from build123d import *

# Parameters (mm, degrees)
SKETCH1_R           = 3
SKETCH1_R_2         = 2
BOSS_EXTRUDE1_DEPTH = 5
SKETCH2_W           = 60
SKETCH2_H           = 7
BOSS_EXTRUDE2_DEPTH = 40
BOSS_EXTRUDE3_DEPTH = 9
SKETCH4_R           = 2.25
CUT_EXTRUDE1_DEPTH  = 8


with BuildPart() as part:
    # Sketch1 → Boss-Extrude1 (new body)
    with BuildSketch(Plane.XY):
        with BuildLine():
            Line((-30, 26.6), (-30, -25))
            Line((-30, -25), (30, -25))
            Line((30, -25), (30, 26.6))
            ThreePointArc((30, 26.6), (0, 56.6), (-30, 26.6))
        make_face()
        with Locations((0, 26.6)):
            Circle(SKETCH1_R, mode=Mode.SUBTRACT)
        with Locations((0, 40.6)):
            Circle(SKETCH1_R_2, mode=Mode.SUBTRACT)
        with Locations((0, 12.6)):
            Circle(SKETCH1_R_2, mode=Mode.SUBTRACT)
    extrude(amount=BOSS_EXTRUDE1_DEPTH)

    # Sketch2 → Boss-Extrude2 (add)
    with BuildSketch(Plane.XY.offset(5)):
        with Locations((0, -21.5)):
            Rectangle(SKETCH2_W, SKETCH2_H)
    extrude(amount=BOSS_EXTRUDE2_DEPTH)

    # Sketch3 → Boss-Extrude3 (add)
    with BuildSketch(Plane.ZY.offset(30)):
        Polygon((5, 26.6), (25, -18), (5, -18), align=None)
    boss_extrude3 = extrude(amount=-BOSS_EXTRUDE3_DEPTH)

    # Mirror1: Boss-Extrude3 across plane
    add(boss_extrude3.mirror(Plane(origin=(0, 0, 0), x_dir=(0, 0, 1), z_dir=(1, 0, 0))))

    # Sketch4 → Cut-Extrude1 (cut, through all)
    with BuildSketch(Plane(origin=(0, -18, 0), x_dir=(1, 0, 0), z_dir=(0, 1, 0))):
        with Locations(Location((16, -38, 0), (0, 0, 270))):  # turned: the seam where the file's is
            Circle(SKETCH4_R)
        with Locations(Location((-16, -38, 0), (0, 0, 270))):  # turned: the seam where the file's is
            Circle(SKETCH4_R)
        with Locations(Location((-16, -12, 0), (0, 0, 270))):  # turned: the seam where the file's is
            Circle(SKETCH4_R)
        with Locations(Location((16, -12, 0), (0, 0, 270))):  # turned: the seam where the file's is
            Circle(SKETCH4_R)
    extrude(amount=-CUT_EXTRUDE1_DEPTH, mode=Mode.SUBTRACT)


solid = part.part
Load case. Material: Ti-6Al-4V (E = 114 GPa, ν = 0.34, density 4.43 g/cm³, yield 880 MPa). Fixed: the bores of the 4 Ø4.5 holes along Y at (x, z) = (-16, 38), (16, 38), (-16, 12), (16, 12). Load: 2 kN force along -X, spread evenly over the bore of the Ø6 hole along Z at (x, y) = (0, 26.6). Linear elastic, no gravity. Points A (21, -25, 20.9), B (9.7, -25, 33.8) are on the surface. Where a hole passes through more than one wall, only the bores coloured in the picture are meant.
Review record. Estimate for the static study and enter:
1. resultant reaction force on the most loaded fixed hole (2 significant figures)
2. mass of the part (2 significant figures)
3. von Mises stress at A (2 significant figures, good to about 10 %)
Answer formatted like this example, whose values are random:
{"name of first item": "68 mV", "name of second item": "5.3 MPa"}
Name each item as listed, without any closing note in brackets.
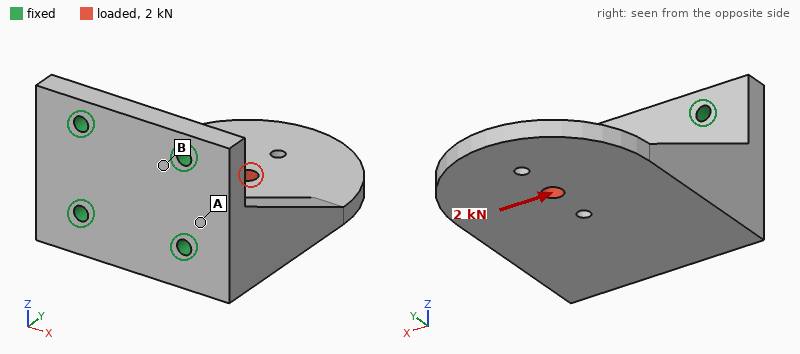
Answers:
{"resultant reaction force on the most loaded fixed hole": "2.8 kN", "mass of the part": "210 g", "von Mises stress at A": "25 MPa"}
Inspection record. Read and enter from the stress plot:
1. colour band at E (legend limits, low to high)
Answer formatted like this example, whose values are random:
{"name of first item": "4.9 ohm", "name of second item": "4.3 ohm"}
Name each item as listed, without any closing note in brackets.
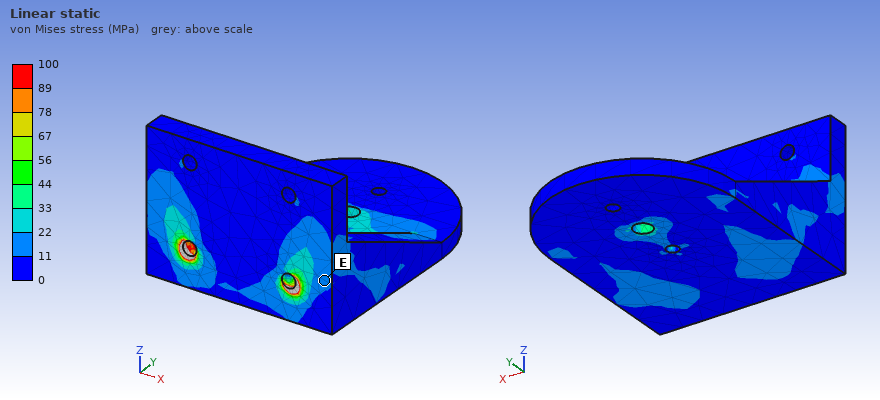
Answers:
{"colour band at E": "11 to 22 MPa"}
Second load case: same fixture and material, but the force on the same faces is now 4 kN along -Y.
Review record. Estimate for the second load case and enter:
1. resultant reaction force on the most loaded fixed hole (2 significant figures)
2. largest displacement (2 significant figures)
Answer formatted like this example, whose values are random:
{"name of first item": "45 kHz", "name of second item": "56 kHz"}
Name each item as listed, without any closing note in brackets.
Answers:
{"resultant reaction force on the most loaded fixed hole": "2.4 kN", "largest displacement": "62 µm"}
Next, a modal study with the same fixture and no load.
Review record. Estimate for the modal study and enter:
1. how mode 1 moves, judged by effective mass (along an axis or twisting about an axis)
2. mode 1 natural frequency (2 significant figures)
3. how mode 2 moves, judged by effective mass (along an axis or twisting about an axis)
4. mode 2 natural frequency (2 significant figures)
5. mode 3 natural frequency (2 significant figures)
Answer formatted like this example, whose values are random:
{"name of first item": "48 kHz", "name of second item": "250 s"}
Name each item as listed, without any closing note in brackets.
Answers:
{"how mode 1 moves, judged by effective mass": "along Z", "mode 1 natural frequency": "1900 Hz", "how mode 2 moves, judged by effective mass": "along X", "mode 2 natural frequency": "3400 Hz", "mode 3 natural frequency": "5600 Hz"}
